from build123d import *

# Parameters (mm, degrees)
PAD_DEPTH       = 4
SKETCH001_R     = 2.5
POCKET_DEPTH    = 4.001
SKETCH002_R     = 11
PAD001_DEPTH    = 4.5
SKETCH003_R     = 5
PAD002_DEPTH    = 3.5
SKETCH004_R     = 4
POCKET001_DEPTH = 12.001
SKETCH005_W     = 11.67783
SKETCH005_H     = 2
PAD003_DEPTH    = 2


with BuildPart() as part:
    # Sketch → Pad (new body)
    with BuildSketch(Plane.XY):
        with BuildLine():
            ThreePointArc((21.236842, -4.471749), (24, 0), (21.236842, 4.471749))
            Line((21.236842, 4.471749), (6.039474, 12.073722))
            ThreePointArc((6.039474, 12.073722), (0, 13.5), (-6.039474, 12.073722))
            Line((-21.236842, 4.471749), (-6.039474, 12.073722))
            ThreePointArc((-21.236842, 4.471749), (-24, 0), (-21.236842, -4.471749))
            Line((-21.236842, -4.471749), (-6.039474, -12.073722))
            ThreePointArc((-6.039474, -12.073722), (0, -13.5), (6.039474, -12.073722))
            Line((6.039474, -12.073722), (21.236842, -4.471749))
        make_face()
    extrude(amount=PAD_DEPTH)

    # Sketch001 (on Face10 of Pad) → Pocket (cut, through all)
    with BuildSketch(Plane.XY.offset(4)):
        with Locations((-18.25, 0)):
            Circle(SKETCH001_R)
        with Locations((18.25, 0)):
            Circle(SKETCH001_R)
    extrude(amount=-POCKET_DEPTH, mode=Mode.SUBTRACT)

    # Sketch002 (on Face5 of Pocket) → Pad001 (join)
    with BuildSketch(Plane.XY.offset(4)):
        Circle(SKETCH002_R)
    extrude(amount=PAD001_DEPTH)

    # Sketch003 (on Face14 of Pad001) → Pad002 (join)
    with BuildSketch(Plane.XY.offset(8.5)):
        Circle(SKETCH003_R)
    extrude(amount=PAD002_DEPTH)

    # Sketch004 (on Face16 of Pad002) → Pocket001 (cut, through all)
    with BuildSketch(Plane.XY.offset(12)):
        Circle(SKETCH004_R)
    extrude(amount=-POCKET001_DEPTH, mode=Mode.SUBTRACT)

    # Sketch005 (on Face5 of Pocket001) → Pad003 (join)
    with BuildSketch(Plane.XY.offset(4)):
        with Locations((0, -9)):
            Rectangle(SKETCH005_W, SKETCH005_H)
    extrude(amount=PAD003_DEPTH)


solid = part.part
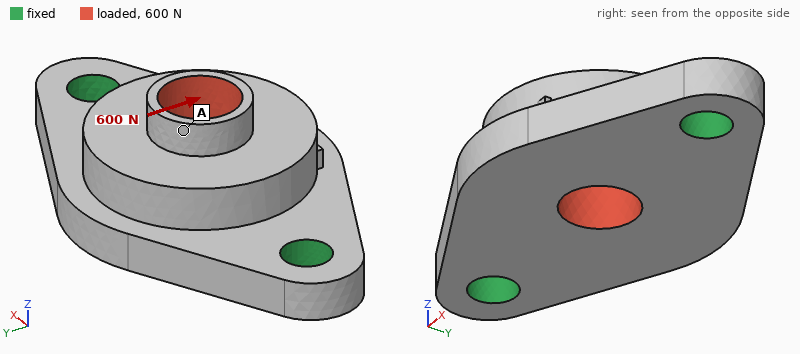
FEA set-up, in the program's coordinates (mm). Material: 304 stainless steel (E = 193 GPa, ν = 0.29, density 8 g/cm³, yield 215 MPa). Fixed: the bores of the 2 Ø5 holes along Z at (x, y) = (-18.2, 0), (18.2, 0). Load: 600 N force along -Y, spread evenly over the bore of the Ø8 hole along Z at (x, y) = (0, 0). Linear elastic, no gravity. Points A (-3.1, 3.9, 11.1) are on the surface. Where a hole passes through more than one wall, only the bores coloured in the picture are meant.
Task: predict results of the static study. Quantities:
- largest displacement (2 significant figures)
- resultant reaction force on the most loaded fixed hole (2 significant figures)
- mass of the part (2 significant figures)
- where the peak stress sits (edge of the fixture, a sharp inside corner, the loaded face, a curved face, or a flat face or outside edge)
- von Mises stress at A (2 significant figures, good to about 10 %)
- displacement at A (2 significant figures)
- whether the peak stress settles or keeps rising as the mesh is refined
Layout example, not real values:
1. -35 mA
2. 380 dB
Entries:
1. 5.5 µm
2. 300 N
3. 37 g
4. edge of the fixture
5. 5.7 MPa
6. 4.8 µm
7. keeps rising
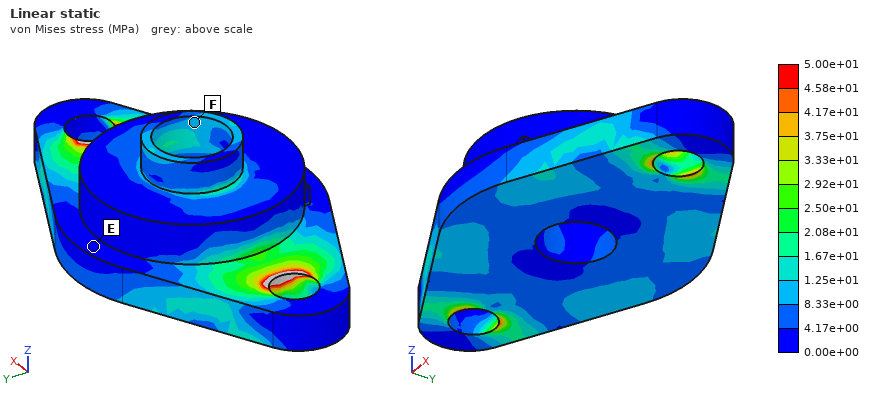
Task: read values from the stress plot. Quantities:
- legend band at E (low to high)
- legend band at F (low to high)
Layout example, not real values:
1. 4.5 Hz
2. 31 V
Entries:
1. 0.00e+00 to 4.17e+00 MPa
2. 8.33e+00 to 1.25e+01 MPa
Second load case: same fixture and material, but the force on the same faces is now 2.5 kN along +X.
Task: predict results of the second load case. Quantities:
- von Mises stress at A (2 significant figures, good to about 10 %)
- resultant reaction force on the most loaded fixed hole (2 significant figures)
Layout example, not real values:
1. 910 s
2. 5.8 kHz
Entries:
1. 23 MPa
2. 1.3 kN
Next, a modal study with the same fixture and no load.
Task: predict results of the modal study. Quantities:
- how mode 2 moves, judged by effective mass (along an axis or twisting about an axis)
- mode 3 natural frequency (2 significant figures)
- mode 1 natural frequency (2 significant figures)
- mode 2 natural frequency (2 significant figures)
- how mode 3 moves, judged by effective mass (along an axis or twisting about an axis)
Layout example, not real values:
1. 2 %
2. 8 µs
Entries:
1. along Z
2. 26 kHz
3. 10 kHz
4. 14 kHz
5. along Y
